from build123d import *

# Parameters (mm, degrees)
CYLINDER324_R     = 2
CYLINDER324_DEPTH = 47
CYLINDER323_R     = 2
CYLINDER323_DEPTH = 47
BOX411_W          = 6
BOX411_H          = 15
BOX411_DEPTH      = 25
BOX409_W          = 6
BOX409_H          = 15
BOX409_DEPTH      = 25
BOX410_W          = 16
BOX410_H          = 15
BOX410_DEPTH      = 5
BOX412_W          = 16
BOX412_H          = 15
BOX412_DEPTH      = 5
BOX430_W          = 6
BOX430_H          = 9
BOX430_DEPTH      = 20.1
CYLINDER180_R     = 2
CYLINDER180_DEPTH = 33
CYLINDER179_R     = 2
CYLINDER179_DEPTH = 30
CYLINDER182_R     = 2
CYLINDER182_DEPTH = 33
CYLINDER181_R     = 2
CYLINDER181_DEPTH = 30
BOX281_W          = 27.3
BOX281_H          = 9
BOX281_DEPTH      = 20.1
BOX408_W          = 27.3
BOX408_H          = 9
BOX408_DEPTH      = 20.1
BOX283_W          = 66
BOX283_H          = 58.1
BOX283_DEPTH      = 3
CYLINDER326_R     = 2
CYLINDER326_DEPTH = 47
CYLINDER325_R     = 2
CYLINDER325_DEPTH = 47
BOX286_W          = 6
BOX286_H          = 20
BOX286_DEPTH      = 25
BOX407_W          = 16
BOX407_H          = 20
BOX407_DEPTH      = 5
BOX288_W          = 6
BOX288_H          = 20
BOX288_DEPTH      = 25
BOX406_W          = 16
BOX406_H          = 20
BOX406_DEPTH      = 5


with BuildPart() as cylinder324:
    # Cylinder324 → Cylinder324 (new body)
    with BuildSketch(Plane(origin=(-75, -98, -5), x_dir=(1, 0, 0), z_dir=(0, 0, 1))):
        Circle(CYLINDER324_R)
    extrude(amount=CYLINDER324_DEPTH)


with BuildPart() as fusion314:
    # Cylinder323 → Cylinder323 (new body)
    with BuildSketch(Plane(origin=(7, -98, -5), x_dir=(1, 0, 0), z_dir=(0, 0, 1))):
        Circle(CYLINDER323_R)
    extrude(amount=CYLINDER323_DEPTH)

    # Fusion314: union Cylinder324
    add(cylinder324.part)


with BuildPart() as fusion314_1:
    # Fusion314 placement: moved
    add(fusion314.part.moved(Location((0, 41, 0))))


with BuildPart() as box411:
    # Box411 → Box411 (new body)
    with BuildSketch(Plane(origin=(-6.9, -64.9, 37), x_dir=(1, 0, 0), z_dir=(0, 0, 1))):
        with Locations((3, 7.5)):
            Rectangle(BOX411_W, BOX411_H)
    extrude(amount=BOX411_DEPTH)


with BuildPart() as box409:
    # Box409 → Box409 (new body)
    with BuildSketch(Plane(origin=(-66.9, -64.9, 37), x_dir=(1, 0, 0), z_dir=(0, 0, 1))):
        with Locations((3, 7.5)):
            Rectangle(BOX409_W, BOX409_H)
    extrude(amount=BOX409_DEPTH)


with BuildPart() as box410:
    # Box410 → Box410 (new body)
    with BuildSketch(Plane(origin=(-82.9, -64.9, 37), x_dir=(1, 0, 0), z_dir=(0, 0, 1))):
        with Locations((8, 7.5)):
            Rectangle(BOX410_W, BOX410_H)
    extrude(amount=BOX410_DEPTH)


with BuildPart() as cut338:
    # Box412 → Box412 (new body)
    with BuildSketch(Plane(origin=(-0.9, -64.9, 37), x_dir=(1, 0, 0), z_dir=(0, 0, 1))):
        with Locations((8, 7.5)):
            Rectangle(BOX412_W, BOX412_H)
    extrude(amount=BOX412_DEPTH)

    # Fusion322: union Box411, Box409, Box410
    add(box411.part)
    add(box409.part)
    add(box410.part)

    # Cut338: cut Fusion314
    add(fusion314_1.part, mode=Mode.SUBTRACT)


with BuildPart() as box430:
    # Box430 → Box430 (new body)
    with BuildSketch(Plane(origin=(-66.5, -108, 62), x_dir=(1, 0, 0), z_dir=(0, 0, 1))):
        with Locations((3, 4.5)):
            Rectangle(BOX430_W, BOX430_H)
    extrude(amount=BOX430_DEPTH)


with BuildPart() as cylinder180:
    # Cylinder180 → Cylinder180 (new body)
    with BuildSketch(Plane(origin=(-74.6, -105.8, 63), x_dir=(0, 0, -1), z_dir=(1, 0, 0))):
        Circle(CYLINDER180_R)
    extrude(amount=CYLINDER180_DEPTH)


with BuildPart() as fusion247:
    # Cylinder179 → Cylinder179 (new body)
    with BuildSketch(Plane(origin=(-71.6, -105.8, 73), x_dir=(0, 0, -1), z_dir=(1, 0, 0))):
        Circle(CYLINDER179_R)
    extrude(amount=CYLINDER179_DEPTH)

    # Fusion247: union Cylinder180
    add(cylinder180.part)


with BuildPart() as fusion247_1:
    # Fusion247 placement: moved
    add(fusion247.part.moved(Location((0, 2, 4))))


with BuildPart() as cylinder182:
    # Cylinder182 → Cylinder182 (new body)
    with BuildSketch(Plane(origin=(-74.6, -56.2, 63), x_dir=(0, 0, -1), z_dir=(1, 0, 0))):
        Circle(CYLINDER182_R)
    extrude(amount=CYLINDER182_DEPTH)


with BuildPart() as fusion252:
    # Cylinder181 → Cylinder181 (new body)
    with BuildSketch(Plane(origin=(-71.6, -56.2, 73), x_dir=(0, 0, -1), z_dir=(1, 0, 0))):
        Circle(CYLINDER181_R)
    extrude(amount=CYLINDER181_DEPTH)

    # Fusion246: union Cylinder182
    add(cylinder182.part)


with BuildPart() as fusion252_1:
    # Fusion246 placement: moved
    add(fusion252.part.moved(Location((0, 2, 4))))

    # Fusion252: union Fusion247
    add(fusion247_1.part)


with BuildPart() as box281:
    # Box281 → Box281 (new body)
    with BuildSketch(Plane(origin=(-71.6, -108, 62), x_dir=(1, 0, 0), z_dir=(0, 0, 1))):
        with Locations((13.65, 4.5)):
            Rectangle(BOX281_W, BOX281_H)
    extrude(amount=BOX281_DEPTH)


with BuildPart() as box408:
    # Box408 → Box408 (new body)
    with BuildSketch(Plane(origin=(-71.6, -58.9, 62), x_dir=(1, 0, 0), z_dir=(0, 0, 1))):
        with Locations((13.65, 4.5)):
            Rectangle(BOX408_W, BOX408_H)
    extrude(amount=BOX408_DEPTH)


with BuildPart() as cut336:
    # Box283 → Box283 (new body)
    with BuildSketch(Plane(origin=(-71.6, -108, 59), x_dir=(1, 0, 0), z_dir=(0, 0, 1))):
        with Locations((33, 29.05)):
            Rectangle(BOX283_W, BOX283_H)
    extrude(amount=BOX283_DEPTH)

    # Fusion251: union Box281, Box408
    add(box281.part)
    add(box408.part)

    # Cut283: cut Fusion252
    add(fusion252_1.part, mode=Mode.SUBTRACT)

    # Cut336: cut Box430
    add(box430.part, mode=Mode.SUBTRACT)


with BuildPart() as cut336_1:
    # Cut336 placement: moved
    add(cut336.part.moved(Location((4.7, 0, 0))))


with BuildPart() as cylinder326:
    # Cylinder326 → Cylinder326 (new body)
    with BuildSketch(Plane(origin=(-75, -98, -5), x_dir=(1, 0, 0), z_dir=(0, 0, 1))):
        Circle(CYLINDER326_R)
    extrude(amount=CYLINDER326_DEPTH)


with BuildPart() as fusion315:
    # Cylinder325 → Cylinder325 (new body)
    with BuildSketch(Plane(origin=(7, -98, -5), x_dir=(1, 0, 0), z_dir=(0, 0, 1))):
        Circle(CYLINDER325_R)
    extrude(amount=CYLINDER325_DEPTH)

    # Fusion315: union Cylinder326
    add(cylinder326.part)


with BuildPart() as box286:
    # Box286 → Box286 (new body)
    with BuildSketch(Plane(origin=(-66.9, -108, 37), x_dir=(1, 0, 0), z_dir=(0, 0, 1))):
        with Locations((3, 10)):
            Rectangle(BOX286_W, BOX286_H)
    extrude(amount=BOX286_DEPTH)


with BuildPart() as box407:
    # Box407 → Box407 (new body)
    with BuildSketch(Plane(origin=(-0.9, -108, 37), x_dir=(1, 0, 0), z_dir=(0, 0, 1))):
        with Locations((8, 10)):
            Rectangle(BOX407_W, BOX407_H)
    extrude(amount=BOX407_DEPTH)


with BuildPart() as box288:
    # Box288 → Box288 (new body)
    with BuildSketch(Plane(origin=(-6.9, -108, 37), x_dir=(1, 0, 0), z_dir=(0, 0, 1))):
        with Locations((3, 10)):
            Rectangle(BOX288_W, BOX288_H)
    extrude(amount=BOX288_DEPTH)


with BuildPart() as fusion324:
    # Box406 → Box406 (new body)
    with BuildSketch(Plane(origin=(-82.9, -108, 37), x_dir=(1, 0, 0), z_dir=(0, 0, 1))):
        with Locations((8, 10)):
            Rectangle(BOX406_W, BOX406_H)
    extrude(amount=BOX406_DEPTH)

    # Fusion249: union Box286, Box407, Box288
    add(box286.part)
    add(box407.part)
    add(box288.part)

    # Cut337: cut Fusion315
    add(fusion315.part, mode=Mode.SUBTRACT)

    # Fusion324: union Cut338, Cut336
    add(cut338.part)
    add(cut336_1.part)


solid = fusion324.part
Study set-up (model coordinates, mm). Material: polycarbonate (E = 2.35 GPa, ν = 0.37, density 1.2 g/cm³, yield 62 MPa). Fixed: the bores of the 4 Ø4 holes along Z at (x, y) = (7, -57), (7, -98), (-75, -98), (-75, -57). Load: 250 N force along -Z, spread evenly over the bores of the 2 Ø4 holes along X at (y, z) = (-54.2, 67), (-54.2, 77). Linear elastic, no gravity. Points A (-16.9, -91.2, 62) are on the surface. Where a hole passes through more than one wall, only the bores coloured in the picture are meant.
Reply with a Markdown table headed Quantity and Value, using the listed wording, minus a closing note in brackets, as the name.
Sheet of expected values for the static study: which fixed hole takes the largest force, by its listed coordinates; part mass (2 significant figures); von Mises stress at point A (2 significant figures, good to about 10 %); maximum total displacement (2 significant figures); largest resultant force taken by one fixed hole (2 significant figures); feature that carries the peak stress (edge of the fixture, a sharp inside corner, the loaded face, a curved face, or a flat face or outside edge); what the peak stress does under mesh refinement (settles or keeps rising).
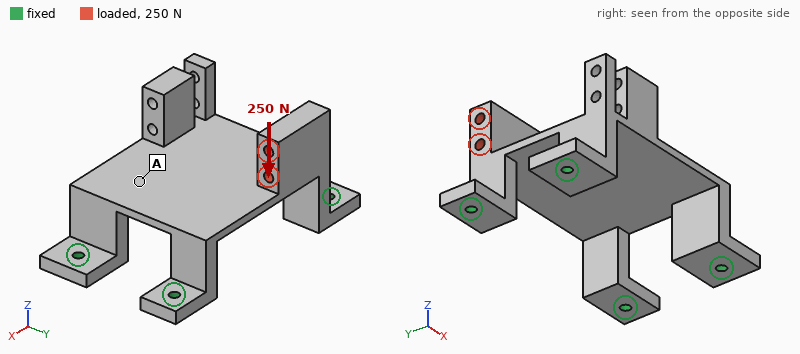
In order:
| Quantity | Value |
|---|---|
| which fixed hole takes the largest force, by its listed coordinates | (-75, -57) |
| part mass | 40 g |
| von Mises stress at point A | 2.2 MPa |
| maximum total displacement | 1.1 mm |
| largest resultant force taken by one fixed hole | 230 N |
| feature that carries the peak stress | edge of the fixture |
| what the peak stress does under mesh refinement | keeps rising |
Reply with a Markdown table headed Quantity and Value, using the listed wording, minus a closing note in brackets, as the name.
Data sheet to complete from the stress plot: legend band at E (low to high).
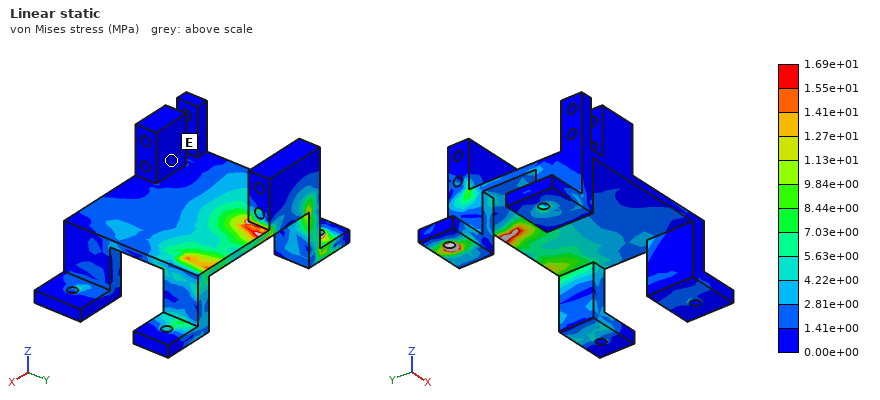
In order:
| Quantity | Value |
|---|---|
| legend band at E | 0.00e+00 to 1.41e+00 MPa |
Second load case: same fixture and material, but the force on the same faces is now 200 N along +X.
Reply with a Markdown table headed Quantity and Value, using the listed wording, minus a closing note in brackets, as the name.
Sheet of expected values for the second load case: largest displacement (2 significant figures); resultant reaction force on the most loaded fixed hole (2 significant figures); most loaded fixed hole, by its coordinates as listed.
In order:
| Quantity | Value |
|---|---|
| largest displacement | 1.4 mm |
| resultant reaction force on the most loaded fixed hole | 96 N |
| most loaded fixed hole, by its coordinates as listed | (7, -57) |
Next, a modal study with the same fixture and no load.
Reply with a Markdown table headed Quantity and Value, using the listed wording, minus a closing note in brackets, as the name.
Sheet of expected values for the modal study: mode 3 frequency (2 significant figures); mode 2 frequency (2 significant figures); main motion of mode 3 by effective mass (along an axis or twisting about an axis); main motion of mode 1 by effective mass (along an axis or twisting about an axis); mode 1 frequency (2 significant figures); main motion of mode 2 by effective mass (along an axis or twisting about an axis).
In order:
| Quantity | Value |
|---|---|
| mode 3 frequency | 960 Hz |
| mode 2 frequency | 680 Hz |
| main motion of mode 3 by effective mass | along Y |
| main motion of mode 1 by effective mass | along Y |
| mode 1 frequency | 640 Hz |
| main motion of mode 2 by effective mass | along X |
